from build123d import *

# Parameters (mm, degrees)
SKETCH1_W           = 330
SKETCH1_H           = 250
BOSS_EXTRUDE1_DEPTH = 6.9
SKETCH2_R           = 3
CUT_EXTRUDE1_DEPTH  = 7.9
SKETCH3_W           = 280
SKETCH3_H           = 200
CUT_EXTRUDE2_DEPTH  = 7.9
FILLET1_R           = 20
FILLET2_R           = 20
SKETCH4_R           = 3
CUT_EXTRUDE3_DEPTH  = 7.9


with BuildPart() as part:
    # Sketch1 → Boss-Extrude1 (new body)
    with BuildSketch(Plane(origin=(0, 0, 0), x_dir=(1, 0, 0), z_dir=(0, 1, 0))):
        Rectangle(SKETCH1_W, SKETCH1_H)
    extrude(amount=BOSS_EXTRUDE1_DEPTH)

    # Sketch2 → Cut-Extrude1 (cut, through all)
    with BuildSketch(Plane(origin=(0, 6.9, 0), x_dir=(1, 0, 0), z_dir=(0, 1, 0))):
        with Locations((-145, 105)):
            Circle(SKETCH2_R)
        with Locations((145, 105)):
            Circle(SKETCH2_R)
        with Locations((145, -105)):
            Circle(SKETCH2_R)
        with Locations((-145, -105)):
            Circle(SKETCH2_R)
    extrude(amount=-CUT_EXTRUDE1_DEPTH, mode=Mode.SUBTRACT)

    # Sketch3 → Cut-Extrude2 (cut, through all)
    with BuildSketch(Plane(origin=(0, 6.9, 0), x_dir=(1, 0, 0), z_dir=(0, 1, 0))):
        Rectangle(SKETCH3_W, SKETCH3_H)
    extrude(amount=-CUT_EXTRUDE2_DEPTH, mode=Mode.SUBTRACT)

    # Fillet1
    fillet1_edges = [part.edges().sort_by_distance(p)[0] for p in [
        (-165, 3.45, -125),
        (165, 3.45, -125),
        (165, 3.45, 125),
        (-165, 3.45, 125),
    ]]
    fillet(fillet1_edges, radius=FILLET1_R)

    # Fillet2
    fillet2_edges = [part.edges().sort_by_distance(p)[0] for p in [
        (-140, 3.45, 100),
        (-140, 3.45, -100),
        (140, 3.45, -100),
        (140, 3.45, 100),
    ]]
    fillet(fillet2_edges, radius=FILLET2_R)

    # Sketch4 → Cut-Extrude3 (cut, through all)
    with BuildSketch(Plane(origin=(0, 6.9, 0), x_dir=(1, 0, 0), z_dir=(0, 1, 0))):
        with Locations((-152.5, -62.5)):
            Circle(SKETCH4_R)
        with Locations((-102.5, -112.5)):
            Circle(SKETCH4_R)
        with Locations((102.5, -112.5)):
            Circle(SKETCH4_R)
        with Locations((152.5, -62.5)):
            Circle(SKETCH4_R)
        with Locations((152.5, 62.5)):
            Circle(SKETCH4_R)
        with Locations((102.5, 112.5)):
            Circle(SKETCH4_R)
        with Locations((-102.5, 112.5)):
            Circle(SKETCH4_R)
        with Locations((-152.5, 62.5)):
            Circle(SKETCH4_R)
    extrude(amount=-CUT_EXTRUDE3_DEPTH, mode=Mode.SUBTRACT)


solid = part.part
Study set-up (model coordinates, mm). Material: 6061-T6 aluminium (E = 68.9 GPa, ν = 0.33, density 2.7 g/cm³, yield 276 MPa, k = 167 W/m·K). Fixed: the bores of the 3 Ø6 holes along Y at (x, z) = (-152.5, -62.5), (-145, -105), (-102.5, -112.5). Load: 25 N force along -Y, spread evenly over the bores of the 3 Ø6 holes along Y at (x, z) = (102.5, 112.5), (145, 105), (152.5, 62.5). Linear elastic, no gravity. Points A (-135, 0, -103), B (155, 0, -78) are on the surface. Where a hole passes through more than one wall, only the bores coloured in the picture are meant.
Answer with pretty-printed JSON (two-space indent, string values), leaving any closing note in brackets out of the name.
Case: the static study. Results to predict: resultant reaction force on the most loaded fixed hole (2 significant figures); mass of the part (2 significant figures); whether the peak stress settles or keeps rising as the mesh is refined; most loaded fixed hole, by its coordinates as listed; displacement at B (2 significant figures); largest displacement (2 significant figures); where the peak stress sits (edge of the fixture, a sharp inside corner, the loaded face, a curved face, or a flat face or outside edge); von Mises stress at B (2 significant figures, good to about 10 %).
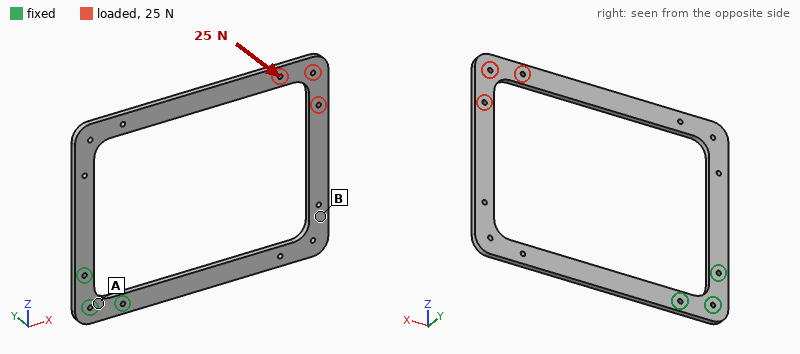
{
  "resultant reaction force on the most loaded fixed hole": "26 N",
  "mass of the part": "490 g",
  "whether the peak stress settles or keeps rising as the mesh is refined": "keeps rising",
  "most loaded fixed hole, by its coordinates as listed": "(-102.5, -112.5)",
  "displacement at B": "2.2 mm",
  "largest displacement": "4.2 mm",
  "where the peak stress sits": "edge of the fixture",
  "von Mises stress at B": "7.5 MPa"
}
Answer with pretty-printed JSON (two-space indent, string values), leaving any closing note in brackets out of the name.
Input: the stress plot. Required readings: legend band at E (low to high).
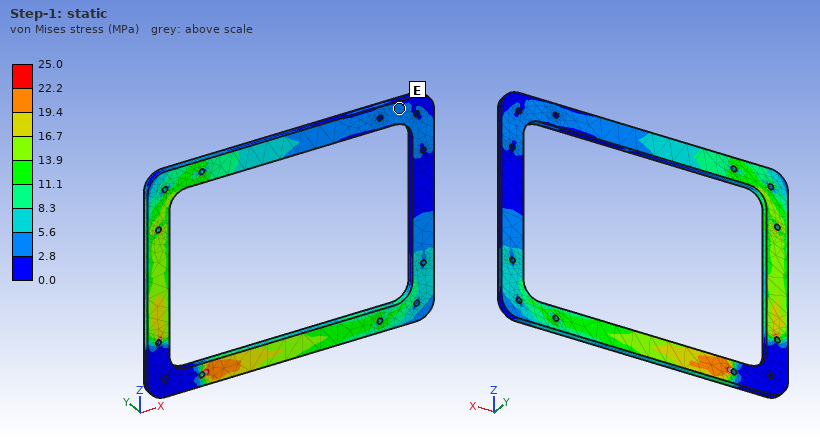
{
  "legend band at E": "2.8 to 5.6 MPa"
}
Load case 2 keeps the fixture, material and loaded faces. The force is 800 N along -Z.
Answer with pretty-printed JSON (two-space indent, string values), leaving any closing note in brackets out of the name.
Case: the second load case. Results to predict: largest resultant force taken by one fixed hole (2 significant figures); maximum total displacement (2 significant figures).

{
  "largest resultant force taken by one fixed hole": "2.3 kN",
  "maximum total displacement": "3.5 mm"
}
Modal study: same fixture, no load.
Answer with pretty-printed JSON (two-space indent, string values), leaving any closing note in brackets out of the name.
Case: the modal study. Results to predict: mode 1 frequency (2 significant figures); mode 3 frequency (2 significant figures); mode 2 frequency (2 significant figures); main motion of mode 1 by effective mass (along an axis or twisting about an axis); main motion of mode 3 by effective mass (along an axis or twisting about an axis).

{
  "mode 1 frequency": "35 Hz",
  "mode 3 frequency": "150 Hz",
  "mode 2 frequency": "80 Hz",
  "main motion of mode 1 by effective mass": "along Y",
  "main motion of mode 3 by effective mass": "along Y"
}
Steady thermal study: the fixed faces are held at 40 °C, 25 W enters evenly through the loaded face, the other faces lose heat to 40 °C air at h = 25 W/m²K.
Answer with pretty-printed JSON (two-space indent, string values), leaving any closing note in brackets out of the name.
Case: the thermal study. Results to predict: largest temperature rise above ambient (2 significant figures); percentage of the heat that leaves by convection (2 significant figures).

{
  "largest temperature rise above ambient": "47 K",
  "percentage of the heat that leaves by convection": "94 %"
}
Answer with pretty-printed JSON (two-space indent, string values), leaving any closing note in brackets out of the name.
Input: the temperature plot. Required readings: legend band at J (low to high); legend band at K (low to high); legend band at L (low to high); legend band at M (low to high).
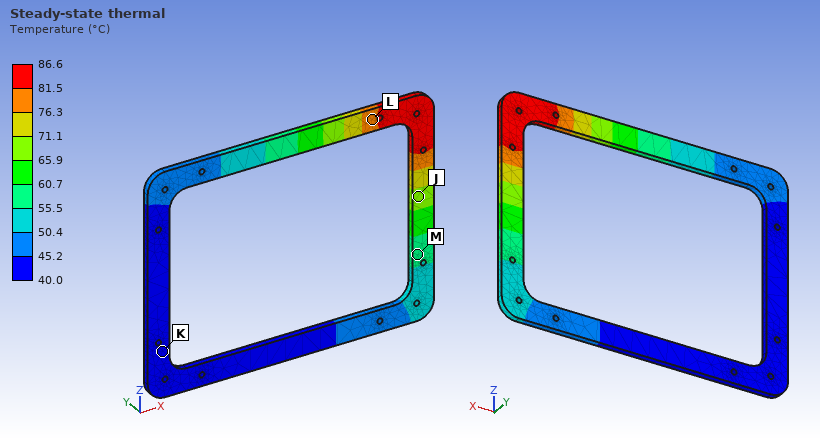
{
  "legend band at J": "65.9 to 71.1 °C",
  "legend band at K": "40.0 to 45.2 °C",
  "legend band at L": "76.3 to 81.5 °C",
  "legend band at M": "55.5 to 60.7 °C"
}
